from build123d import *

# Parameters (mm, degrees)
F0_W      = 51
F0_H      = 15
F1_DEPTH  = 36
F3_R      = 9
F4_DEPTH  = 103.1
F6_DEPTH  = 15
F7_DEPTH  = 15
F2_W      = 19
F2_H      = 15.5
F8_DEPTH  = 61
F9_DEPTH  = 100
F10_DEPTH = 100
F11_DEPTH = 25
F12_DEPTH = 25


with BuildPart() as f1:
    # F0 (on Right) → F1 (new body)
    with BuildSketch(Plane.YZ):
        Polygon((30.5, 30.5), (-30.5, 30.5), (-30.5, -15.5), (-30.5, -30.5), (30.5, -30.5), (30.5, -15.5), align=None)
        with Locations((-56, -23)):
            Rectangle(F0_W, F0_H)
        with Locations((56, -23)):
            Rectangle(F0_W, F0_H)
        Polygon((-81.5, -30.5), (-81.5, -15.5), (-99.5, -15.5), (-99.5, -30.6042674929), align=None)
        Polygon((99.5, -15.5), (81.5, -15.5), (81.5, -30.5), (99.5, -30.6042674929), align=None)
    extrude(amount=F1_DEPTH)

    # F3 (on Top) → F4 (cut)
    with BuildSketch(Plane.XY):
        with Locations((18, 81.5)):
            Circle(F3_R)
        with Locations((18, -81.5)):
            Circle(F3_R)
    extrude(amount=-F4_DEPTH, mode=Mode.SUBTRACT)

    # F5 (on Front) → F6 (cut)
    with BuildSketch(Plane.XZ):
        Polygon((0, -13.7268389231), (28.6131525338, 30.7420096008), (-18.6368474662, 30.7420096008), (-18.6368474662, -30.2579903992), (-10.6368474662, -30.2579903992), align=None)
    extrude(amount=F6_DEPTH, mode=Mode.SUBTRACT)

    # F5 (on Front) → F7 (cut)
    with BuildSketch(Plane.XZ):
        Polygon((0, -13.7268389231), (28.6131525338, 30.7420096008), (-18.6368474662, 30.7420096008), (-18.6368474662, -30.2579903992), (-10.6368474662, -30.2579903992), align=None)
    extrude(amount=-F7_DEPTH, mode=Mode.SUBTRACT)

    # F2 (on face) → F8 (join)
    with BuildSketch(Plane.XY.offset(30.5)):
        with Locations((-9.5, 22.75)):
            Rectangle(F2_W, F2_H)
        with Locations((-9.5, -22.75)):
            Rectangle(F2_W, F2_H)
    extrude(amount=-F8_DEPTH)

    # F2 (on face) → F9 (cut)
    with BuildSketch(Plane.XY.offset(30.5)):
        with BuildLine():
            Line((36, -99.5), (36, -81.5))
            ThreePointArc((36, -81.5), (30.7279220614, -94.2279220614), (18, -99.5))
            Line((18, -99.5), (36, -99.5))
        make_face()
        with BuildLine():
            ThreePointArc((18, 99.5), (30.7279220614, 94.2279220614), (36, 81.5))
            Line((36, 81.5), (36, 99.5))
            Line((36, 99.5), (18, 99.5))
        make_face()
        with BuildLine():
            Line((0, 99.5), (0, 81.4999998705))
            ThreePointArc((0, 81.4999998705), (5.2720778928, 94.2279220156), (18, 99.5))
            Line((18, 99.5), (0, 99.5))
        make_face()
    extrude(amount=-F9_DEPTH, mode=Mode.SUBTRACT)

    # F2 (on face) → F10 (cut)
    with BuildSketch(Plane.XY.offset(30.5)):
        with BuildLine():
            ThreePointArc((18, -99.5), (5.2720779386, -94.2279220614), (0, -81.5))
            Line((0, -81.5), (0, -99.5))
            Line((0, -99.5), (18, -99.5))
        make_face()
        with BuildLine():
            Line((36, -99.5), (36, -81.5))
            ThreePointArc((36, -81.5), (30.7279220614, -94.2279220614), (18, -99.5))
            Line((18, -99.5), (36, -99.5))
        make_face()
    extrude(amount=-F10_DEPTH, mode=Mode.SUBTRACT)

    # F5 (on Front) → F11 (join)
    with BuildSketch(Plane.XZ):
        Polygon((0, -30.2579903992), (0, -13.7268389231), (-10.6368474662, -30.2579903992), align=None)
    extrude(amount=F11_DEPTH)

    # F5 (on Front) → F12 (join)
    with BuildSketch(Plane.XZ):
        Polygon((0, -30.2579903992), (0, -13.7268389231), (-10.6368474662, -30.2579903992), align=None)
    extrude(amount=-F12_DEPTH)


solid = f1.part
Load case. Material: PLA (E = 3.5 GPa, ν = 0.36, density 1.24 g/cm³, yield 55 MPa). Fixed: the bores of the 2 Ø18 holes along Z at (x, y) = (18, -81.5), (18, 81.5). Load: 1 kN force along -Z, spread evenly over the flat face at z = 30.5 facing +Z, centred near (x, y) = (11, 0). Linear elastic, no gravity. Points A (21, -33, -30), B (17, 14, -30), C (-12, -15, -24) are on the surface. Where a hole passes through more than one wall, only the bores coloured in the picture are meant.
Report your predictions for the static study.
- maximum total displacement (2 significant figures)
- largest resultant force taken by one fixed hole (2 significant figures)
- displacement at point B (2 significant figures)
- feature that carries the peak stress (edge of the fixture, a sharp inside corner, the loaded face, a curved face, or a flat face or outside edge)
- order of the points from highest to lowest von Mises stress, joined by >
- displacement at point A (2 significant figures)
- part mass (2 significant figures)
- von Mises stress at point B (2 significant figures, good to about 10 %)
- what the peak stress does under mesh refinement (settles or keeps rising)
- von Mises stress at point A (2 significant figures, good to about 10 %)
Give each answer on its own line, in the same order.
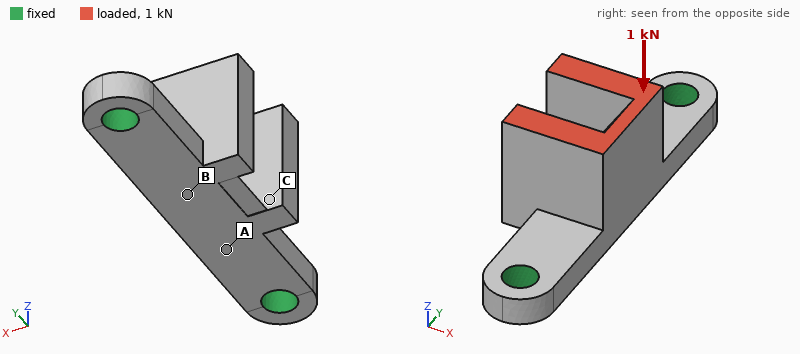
0.41 mm
550 N
0.21 mm
edge of the fixture
A > B > C
0.17 mm
270 g
2.4 MPa
keeps rising
4.4 MPa
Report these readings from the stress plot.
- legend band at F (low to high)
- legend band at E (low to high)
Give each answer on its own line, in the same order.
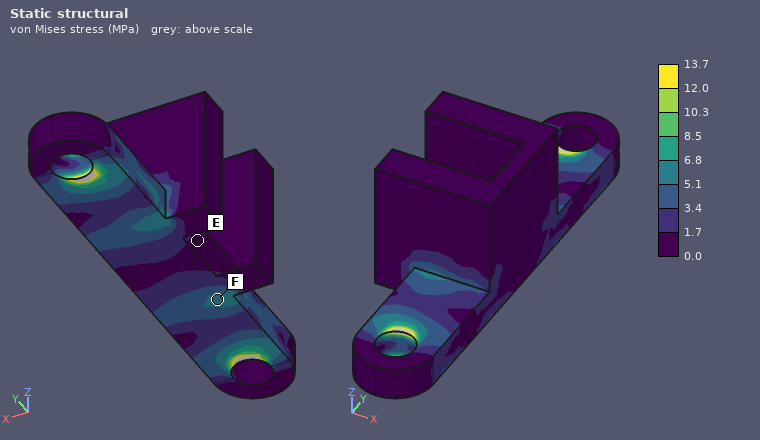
5.1 to 6.8 MPa
0.0 to 1.7 MPa
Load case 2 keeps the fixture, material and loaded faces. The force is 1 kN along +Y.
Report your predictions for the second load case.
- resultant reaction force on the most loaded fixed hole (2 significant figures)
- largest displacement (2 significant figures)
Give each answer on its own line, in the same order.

700 N
0.38 mm
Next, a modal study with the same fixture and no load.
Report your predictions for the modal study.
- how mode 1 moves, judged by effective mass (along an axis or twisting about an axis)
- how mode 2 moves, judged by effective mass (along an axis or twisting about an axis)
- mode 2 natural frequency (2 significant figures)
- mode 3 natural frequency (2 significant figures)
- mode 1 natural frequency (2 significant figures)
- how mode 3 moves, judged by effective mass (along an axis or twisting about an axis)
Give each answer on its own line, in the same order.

along X
along Z
770 Hz
1200 Hz
460 Hz
along Y
